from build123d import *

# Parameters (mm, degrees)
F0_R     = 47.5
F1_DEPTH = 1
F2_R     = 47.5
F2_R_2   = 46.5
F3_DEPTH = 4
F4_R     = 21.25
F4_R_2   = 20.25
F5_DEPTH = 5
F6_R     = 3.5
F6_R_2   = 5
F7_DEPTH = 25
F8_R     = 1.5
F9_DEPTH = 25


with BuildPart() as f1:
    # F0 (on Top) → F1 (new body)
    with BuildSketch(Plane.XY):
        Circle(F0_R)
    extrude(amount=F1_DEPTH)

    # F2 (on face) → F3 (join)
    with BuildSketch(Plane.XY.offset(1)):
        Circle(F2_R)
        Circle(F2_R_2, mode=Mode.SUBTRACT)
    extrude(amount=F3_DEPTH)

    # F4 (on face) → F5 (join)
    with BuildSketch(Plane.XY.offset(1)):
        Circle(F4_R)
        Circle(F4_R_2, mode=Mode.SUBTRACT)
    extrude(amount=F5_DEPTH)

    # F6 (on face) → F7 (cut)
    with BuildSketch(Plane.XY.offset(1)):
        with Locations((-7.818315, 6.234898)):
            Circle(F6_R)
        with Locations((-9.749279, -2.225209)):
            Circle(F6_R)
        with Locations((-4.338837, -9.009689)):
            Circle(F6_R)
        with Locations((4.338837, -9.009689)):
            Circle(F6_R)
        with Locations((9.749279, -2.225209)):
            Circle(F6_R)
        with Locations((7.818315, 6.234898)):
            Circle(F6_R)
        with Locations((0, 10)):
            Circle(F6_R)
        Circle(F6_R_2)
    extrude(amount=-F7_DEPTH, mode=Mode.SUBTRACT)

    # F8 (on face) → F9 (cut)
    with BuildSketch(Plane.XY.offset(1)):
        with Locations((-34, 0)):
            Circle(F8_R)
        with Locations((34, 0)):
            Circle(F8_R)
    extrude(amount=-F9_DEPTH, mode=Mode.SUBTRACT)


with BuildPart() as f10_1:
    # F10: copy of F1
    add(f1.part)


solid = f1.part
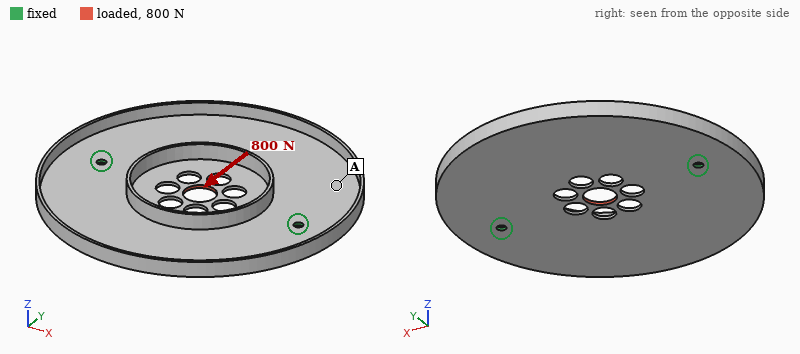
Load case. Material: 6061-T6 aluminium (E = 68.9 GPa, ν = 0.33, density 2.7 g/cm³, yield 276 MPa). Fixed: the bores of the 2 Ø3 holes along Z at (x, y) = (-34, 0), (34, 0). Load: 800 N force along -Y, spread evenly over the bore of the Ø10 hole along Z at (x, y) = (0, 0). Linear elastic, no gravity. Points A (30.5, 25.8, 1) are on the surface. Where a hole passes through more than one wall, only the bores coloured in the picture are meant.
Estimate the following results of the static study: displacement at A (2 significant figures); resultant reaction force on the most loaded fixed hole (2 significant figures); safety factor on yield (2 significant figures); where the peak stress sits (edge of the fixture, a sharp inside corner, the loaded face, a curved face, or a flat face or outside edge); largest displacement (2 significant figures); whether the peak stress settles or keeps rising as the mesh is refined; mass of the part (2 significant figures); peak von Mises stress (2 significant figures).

5.5 µm
400 N
2.0
a curved face
23 µm
settles
23 g
140 MPa
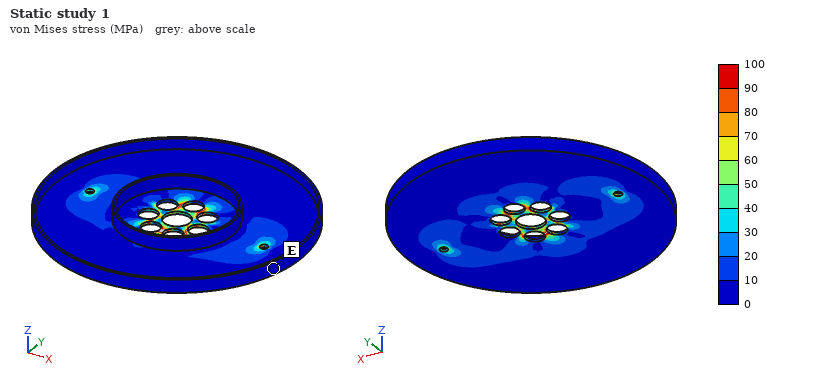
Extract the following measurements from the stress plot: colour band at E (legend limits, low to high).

0 to 10 MPa
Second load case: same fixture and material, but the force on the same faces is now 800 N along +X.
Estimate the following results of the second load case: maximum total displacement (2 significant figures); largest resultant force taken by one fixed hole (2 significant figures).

20 µm
400 N
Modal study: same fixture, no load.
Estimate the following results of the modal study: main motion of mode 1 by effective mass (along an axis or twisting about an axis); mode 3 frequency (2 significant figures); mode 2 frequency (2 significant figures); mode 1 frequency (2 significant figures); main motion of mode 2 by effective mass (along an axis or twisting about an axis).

twisting about X
1200 Hz
780 Hz
390 Hz
along Z
